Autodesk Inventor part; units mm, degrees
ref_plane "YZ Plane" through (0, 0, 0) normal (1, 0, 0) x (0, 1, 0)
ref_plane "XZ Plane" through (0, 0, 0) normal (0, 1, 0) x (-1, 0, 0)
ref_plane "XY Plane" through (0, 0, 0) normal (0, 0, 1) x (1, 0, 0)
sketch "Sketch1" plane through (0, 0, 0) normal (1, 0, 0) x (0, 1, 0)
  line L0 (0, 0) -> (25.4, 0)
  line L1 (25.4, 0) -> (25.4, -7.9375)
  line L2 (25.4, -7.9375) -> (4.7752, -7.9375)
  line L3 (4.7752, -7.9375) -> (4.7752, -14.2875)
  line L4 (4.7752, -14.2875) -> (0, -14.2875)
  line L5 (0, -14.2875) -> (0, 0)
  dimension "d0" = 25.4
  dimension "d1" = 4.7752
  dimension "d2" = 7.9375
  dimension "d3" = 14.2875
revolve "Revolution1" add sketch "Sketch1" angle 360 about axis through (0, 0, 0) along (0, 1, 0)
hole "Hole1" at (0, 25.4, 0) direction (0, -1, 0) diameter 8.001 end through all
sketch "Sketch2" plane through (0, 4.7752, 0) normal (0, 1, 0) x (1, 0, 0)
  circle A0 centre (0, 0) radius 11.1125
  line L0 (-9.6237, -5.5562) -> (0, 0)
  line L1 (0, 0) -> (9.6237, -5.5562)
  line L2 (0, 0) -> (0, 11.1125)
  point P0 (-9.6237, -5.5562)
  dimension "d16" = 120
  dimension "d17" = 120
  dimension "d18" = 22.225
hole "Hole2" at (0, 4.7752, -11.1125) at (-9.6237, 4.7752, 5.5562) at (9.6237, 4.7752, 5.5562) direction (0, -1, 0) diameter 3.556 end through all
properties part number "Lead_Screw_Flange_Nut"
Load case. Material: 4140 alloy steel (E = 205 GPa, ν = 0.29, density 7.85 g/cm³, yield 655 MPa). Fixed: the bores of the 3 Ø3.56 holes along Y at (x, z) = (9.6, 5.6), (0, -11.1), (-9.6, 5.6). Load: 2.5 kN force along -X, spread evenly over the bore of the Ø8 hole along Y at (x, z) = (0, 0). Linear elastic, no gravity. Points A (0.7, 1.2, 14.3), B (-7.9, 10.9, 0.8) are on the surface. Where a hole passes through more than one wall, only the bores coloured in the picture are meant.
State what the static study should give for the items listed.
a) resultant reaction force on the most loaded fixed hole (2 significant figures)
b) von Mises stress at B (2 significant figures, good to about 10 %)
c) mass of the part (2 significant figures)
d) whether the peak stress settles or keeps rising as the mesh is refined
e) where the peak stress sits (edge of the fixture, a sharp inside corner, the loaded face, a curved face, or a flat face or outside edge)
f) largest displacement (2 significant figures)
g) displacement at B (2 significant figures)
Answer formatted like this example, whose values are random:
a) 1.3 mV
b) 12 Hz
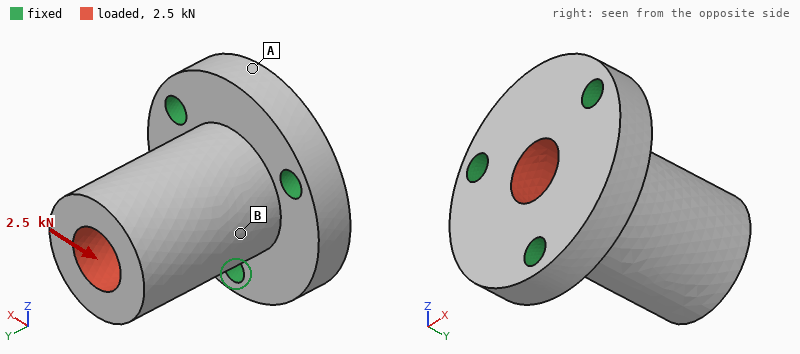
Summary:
a) 1.6 kN
b) 26 MPa
c) 45 g
d) keeps rising
e) edge of the fixture
f) 15 µm
g) 6.2 µm
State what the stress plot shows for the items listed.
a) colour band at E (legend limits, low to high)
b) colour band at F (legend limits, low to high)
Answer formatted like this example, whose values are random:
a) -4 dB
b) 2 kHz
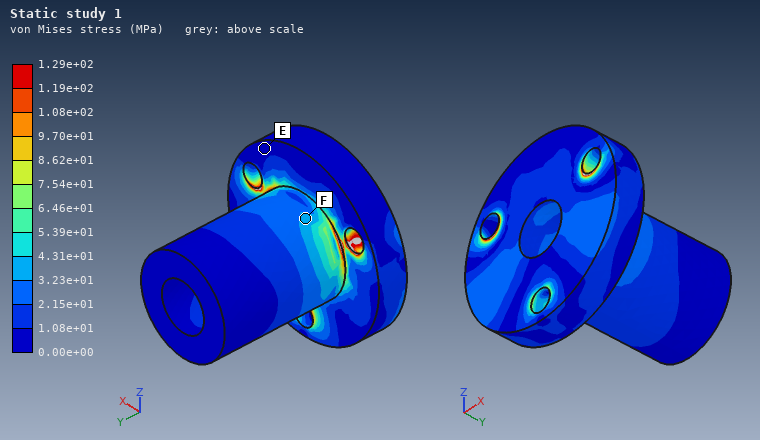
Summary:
a) 0.00e+00 to 1.08e+01 MPa
b) 3.23e+01 to 4.31e+01 MPa
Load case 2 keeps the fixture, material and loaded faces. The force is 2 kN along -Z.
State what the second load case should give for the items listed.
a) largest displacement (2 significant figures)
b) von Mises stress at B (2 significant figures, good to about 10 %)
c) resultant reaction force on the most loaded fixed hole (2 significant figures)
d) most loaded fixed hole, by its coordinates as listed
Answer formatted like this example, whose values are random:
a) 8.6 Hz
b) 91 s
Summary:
a) 12 µm
b) 18 MPa
c) 1.5 kN
d) (0, -11.1)
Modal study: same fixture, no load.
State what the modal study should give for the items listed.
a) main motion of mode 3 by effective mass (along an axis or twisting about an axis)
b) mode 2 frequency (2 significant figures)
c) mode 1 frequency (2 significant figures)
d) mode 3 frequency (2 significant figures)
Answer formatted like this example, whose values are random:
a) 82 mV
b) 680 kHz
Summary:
a) along Y
b) 14 kHz
c) 14 kHz
d) 32 kHz
